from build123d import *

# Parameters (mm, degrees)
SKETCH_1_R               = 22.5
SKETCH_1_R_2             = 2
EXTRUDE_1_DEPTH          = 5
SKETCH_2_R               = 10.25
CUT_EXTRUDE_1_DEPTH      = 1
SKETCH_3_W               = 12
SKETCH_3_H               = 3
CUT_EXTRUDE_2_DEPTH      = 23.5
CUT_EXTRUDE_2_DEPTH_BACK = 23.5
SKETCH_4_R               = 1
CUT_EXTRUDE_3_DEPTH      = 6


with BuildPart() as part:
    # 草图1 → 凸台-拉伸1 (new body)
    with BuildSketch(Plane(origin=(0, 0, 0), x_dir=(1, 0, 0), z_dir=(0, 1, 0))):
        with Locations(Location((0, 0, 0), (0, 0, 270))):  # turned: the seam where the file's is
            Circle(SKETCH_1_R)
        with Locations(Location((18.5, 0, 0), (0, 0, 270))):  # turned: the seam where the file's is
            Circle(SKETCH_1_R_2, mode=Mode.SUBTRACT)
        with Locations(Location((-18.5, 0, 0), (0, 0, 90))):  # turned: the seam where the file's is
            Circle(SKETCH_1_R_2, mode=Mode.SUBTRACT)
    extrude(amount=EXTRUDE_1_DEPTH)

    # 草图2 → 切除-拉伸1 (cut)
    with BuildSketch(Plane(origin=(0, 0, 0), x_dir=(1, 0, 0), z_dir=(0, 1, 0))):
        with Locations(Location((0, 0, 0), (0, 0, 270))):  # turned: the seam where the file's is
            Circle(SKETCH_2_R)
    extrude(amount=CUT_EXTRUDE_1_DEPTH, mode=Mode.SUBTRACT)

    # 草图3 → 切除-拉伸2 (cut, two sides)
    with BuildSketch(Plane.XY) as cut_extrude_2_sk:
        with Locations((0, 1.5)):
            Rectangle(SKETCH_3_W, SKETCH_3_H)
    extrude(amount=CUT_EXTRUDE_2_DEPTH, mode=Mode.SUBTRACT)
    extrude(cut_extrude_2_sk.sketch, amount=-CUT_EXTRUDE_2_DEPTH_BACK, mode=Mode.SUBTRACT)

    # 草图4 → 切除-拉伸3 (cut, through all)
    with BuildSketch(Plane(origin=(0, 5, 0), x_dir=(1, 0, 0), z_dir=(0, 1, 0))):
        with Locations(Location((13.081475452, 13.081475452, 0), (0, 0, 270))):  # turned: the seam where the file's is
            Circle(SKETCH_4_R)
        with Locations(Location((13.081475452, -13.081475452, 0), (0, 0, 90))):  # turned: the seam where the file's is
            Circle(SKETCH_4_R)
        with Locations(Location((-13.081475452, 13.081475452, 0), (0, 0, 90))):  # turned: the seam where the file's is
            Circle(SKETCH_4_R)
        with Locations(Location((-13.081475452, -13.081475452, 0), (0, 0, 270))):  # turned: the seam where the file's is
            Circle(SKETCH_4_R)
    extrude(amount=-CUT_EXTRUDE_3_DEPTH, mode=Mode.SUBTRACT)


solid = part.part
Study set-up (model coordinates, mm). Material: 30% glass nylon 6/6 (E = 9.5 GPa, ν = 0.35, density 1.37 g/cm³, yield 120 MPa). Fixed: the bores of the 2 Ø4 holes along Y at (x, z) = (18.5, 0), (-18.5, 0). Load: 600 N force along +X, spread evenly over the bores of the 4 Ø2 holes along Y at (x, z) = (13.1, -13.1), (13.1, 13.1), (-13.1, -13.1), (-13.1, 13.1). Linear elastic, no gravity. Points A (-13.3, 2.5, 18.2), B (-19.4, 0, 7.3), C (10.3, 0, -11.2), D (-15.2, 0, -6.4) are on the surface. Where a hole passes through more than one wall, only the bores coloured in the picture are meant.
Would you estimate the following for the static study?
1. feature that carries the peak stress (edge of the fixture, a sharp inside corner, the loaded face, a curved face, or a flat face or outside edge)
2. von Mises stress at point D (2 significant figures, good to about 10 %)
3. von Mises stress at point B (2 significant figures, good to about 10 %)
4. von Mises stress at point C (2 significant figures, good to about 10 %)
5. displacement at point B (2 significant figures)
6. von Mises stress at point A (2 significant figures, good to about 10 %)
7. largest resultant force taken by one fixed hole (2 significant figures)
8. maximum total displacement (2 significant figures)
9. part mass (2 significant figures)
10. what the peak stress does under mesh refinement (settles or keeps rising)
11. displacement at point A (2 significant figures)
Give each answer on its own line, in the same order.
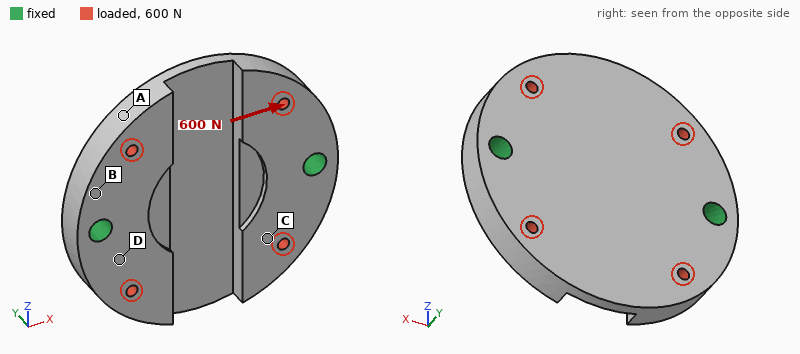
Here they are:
edge of the fixture
3.6 MPa
2.0 MPa
4.2 MPa
5.5 µm
0.86 MPa
300 N
14 µm
8.3 g
keeps rising
13 µm
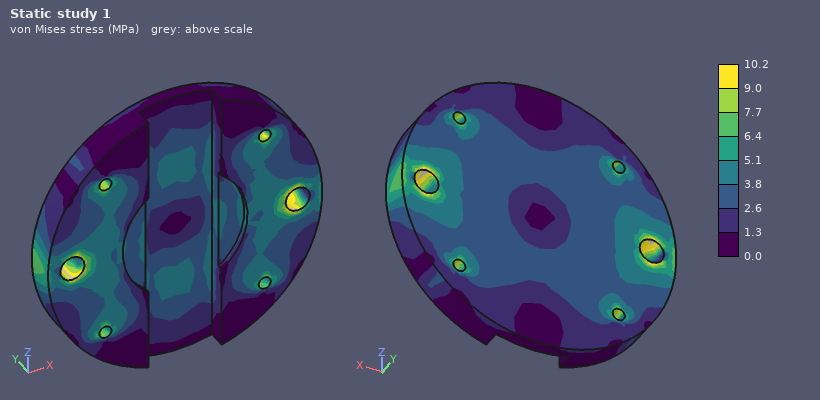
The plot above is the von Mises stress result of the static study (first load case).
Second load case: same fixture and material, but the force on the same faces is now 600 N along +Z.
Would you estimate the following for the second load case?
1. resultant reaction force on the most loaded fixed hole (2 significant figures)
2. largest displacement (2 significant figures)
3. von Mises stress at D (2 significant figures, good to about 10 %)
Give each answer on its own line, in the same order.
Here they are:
300 N
11 µm
3.8 MPa
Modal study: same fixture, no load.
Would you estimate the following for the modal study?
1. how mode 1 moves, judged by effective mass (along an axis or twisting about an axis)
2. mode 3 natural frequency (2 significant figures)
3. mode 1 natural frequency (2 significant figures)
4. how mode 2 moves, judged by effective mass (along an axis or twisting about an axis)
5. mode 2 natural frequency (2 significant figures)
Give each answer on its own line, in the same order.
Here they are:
twisting about X
7100 Hz
3900 Hz
along Y
4900 Hz
